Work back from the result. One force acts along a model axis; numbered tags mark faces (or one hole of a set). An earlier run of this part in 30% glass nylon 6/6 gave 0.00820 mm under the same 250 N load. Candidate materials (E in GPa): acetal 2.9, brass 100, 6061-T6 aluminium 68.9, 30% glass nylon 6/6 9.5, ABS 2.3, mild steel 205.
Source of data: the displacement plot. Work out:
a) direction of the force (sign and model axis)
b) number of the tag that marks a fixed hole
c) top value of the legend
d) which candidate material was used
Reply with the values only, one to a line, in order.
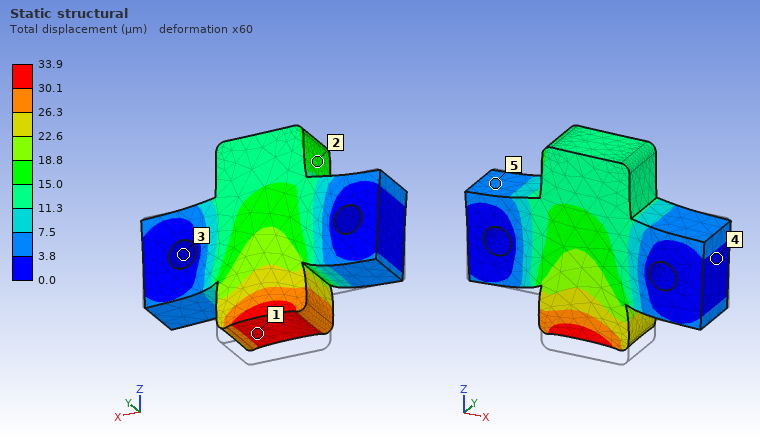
+Z
3
33.9 µm
ABS
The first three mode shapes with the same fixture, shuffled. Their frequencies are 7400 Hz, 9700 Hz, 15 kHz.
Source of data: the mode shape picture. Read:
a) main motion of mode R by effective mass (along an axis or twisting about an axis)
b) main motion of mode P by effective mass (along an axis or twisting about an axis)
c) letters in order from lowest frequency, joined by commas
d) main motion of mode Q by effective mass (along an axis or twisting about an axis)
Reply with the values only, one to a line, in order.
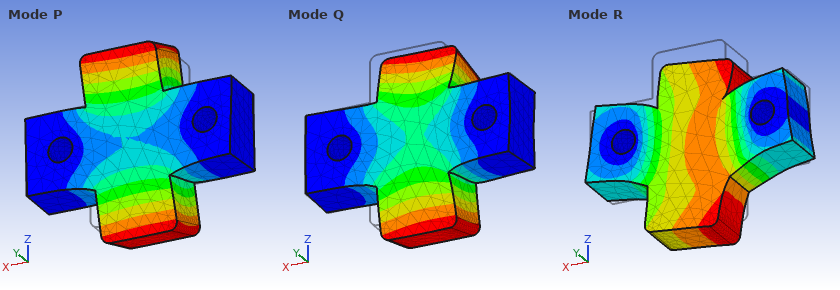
along Z
twisting about X
P, Q, R
along Y
